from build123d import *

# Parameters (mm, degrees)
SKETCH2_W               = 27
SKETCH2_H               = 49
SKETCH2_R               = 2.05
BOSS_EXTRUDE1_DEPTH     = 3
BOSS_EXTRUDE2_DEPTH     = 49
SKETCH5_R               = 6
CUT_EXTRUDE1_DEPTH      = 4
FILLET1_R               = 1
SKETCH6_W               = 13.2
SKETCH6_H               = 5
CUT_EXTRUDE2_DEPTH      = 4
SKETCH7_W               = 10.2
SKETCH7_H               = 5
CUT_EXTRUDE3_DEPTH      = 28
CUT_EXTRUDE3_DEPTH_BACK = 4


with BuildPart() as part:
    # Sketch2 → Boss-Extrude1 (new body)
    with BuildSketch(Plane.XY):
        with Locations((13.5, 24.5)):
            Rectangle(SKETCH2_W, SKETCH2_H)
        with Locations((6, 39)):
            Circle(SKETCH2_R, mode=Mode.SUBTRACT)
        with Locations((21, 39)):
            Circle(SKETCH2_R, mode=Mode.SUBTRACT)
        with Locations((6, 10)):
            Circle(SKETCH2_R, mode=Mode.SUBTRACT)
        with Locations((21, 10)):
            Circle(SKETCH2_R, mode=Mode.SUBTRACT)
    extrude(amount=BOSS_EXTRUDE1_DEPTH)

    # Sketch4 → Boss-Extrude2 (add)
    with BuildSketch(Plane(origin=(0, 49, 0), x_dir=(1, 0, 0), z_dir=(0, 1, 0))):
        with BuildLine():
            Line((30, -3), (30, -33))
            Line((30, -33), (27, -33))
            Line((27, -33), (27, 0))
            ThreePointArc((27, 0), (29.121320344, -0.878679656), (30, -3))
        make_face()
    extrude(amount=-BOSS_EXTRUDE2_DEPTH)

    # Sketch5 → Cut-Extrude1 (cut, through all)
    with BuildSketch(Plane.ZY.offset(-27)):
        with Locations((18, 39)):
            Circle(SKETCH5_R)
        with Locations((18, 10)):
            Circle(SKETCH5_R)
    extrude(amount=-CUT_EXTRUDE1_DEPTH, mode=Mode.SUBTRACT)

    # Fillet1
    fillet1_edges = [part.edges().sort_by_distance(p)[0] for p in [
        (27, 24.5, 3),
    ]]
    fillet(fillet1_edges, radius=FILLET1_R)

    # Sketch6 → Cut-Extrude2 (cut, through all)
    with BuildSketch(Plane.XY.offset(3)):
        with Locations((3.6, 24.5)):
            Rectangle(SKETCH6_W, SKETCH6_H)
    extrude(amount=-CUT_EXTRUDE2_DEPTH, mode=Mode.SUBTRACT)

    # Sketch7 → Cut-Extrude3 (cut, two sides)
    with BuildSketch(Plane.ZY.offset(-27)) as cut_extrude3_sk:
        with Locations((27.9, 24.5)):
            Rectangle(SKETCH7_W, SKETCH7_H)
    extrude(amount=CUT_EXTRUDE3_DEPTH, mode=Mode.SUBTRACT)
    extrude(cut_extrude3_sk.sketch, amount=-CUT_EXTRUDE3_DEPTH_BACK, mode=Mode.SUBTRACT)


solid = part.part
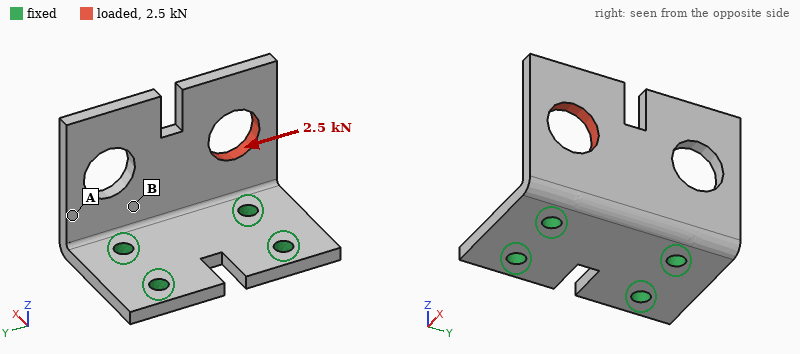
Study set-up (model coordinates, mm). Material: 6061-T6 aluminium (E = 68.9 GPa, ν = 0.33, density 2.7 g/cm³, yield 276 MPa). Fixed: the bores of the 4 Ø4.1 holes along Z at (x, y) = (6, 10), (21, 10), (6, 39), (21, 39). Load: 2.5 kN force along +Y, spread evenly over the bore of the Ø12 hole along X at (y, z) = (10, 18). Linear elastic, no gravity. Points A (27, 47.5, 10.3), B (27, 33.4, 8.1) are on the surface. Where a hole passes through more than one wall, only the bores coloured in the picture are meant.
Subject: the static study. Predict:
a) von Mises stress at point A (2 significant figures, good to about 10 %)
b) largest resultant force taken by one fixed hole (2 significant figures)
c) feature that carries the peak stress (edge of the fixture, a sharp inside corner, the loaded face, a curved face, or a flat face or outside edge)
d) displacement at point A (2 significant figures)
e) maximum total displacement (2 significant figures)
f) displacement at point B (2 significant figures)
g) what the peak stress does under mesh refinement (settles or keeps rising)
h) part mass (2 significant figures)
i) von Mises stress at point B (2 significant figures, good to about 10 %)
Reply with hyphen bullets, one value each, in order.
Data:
- 42 MPa
- 1.9 kN
- edge of the fixture
- 0.090 mm
- 0.22 mm
- 0.046 mm
- keeps rising
- 21 g
- 95 MPa
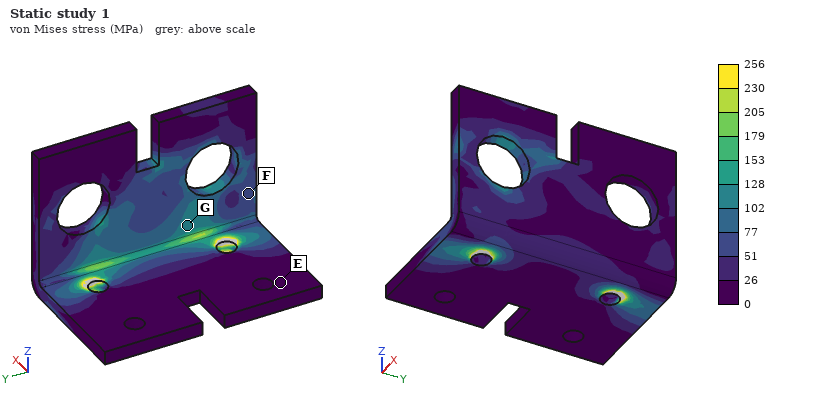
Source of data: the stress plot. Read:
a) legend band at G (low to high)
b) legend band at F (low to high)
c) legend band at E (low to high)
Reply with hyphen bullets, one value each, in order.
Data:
- 102 to 128 MPa
- 51 to 77 MPa
- 0 to 26 MPa
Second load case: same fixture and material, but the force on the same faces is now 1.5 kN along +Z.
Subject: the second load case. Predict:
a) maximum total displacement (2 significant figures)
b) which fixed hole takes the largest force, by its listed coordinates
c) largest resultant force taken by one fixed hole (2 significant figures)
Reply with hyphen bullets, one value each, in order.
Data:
- 0.27 mm
- (21, 10)
- 1.6 kN
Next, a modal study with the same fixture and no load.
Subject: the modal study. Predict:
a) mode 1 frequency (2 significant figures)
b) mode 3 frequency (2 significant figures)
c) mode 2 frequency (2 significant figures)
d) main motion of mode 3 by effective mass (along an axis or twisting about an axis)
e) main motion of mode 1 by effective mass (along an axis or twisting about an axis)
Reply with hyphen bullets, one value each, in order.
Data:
- 2000 Hz
- 7500 Hz
- 3200 Hz
- along Y
- along X
